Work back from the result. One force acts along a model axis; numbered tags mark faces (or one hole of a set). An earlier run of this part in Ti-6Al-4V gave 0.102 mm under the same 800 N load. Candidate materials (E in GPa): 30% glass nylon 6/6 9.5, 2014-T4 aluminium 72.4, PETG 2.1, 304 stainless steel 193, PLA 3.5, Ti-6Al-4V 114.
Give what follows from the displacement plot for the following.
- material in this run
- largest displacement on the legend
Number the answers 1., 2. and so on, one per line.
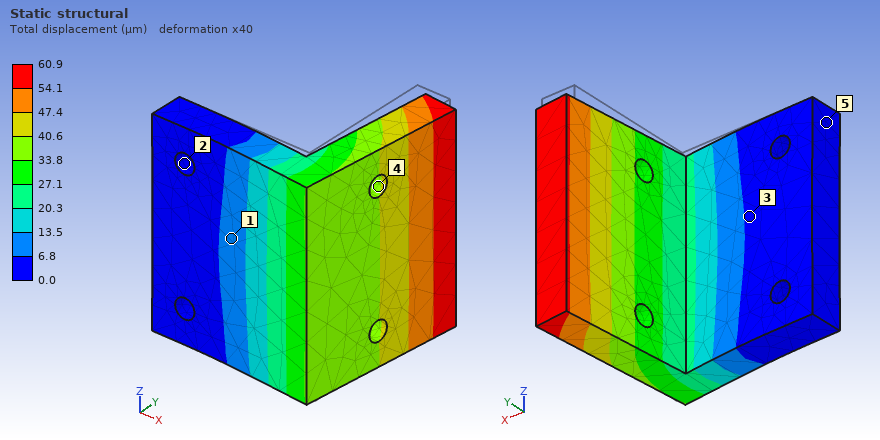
1. 304 stainless steel
2. 60.9 µm
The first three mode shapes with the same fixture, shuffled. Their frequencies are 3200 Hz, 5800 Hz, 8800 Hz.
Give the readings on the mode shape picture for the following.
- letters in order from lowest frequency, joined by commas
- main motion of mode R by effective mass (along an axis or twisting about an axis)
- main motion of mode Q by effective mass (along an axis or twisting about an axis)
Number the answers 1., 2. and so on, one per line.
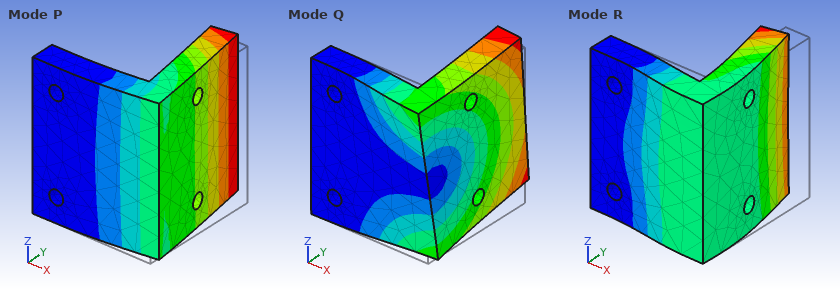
1. P, Q, R
2. along Y
3. along Z
